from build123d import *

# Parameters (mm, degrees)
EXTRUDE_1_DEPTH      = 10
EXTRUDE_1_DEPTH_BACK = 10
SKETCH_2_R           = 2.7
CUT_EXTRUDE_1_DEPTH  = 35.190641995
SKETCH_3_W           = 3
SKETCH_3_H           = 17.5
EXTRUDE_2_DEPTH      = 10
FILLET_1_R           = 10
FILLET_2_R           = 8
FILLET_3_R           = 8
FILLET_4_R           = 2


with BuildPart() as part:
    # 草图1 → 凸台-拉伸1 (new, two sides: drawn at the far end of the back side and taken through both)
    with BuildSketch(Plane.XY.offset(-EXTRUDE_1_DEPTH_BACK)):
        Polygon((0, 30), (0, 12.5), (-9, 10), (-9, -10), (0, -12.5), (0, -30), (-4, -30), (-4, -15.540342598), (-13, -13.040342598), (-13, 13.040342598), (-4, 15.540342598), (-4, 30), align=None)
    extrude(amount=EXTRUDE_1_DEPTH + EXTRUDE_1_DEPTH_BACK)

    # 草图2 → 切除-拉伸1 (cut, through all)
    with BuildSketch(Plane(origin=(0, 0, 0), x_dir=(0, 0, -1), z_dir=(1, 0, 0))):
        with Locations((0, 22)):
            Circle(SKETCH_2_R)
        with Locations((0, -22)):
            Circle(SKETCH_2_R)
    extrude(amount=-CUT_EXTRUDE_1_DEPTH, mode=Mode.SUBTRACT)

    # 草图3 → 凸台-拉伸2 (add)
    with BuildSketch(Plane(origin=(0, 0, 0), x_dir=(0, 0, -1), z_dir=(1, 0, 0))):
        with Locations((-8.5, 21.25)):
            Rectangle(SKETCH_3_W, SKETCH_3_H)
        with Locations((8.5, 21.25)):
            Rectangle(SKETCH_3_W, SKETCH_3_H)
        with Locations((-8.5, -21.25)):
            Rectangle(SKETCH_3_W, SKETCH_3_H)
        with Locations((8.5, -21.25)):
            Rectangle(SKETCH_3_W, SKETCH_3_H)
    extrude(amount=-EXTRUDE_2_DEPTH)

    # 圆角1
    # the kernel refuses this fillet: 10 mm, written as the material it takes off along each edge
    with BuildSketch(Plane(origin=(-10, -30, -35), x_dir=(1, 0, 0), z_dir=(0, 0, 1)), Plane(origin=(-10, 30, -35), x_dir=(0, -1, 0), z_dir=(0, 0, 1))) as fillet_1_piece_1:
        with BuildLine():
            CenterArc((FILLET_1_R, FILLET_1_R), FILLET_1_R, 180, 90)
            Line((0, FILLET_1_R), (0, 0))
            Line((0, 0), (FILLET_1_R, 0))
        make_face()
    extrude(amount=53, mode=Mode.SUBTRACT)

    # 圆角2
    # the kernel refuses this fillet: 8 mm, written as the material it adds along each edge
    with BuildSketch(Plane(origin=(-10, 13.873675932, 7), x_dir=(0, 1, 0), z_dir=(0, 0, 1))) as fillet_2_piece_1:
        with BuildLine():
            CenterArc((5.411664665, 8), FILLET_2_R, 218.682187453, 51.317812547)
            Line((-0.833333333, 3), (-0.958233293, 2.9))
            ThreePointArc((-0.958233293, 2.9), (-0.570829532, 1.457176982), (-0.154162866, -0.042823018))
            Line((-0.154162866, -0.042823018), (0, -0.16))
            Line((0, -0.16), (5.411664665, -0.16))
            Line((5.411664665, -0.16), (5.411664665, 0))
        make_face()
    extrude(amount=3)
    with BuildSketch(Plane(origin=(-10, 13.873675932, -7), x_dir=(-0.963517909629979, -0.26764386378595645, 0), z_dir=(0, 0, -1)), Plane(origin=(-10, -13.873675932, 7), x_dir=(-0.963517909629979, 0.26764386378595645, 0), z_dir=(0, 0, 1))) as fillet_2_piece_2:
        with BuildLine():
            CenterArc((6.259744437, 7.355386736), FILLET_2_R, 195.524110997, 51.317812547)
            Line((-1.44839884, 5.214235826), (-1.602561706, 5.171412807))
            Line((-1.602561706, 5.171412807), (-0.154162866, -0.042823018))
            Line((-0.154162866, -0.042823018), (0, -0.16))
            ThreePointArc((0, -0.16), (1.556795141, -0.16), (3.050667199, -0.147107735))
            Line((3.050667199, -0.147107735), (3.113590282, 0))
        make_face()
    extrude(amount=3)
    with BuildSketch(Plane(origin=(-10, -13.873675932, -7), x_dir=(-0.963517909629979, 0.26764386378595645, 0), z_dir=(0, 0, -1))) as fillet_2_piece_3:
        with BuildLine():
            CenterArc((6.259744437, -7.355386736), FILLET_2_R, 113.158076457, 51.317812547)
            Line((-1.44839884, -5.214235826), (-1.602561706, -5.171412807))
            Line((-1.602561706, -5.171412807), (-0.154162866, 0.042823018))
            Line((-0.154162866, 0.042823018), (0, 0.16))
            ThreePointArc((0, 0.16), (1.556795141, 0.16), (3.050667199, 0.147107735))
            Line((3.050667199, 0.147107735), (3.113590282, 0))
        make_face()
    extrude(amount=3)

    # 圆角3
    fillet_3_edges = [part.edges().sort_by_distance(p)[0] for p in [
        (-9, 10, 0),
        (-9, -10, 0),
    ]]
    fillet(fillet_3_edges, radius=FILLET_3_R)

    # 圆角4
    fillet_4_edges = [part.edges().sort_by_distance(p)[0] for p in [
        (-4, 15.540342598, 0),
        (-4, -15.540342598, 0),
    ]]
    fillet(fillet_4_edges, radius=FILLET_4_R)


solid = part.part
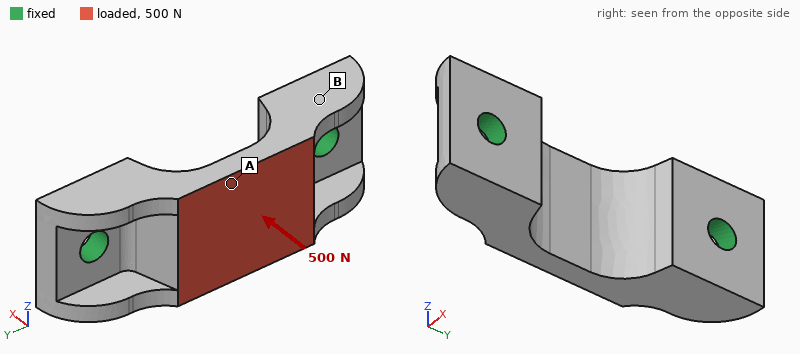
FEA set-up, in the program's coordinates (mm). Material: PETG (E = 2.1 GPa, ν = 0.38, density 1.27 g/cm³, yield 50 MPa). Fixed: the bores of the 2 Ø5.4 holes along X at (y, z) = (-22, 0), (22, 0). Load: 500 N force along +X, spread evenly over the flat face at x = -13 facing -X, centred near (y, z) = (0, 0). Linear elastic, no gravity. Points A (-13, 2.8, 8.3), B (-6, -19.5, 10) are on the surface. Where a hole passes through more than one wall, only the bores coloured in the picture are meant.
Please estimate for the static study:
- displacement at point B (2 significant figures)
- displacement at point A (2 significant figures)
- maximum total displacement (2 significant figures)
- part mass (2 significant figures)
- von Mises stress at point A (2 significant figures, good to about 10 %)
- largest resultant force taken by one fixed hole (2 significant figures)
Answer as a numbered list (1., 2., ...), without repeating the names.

1. 0.045 mm
2. 0.14 mm
3. 0.15 mm
4. 8.7 g
5. 7.8 MPa
6. 380 N
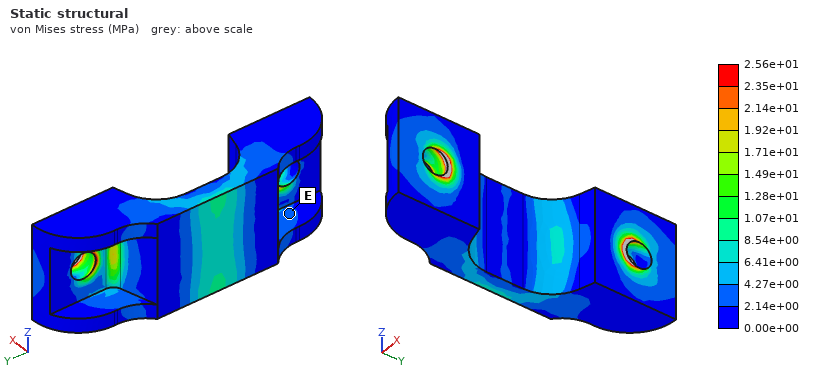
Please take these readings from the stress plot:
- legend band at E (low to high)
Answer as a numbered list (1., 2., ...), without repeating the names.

1. 2.14e+00 to 4.27e+00 MPa
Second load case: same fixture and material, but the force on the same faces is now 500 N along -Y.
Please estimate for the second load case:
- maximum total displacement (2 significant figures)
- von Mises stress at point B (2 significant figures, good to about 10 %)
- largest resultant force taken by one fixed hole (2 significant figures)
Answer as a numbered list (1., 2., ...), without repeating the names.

1. 85 µm
2. 1.6 MPa
3. 280 N
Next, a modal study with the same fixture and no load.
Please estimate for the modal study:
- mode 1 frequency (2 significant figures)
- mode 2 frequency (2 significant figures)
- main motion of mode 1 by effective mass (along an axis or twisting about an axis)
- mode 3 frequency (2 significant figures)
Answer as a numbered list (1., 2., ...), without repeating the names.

1. 2500 Hz
2. 4900 Hz
3. along Z
4. 5000 Hz
